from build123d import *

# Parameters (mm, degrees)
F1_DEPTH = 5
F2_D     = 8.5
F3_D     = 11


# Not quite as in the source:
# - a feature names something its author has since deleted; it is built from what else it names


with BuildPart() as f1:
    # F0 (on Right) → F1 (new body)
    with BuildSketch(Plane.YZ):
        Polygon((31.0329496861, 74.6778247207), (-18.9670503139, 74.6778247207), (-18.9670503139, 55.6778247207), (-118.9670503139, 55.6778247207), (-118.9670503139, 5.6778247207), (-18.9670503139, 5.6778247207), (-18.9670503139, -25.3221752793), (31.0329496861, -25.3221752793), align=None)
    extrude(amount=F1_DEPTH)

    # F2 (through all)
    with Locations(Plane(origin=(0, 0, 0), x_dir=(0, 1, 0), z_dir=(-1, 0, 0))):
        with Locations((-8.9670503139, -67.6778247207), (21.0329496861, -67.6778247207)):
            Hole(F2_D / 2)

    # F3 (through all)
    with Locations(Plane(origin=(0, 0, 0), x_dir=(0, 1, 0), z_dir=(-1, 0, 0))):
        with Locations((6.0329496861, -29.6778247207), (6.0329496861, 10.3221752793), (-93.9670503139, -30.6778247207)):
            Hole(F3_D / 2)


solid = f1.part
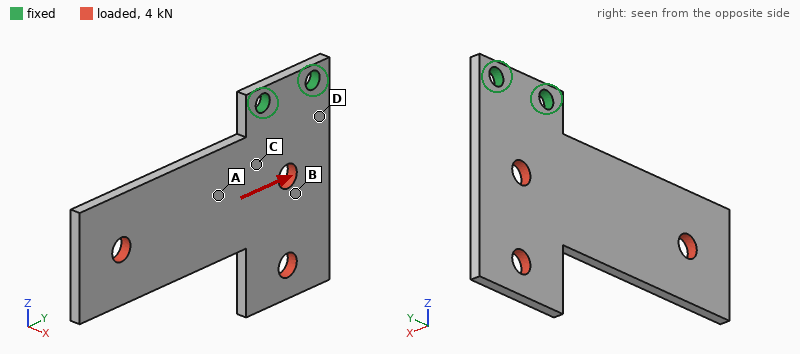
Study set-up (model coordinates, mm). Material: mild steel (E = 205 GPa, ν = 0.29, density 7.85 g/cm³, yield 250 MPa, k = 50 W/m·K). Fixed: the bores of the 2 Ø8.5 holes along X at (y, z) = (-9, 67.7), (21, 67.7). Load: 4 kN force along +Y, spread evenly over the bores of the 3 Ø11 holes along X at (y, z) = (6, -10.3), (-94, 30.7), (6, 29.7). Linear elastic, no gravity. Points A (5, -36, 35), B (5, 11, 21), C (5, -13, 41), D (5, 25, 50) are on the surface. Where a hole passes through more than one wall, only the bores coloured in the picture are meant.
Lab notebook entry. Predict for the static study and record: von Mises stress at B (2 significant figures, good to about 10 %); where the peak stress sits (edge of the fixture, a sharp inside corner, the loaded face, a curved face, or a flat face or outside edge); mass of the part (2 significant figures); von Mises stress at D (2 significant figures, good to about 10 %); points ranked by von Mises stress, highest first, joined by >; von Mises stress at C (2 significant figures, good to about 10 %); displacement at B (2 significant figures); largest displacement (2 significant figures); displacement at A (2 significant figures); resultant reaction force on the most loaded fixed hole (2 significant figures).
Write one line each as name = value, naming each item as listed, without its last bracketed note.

von Mises stress at B = 22 MPa
where the peak stress sits = edge of the fixture
mass of the part = 380 g
von Mises stress at D = 49 MPa
points ranked by von Mises stress, highest first, joined by > = D > C > B > A
von Mises stress at C = 38 MPa
displacement at B = 25 µm
largest displacement = 78 µm
displacement at A = 27 µm
resultant reaction force on the most loaded fixed hole = 6.0 kN
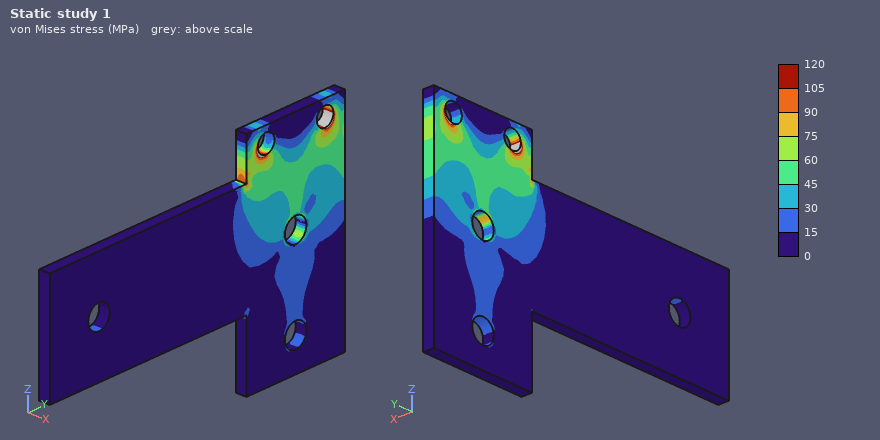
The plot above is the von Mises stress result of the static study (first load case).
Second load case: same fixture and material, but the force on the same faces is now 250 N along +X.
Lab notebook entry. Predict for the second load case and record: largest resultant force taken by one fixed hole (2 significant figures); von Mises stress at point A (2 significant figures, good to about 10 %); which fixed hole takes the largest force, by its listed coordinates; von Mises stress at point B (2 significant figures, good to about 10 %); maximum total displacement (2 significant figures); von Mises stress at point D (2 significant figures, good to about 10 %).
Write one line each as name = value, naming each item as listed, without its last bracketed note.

largest resultant force taken by one fixed hole = 330 N
von Mises stress at point A = 21 MPa
which fixed hole takes the largest force, by its listed coordinates = (-9, 67.7)
von Mises stress at point B = 17 MPa
maximum total displacement = 0.44 mm
von Mises stress at point D = 33 MPa
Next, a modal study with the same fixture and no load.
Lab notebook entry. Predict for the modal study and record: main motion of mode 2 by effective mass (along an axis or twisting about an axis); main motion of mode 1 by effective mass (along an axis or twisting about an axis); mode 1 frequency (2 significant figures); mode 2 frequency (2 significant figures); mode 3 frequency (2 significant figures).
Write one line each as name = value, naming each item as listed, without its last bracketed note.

main motion of mode 2 by effective mass = along X
main motion of mode 1 by effective mass = along X
mode 1 frequency = 270 Hz
mode 2 frequency = 510 Hz
mode 3 frequency = 1400 Hz
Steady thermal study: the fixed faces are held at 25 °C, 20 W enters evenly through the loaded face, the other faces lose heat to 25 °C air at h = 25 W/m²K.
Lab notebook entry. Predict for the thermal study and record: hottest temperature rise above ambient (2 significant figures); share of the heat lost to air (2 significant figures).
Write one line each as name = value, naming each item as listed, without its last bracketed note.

hottest temperature rise above ambient = 38 K
share of the heat lost to air = 60 %
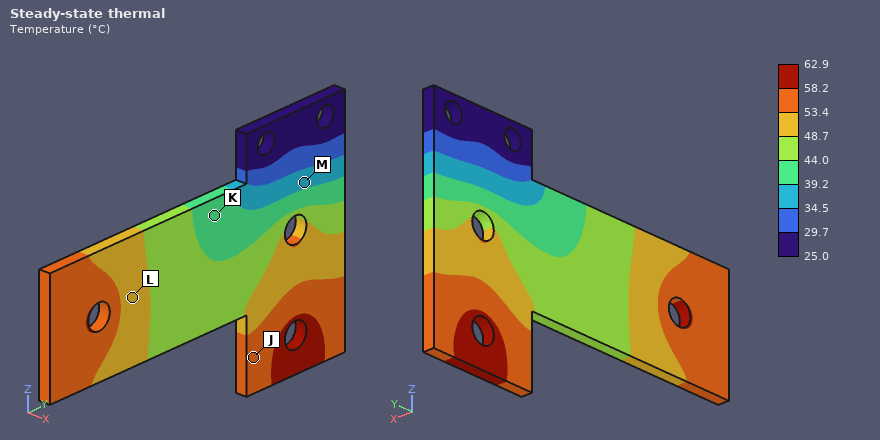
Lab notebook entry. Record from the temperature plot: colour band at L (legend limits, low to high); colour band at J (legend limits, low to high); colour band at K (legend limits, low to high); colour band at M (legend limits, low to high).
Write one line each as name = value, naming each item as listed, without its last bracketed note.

colour band at L = 48.7 to 53.4 °C
colour band at J = 53.4 to 58.2 °C
colour band at K = 39.2 to 44.0 °C
colour band at M = 34.5 to 39.2 °C
